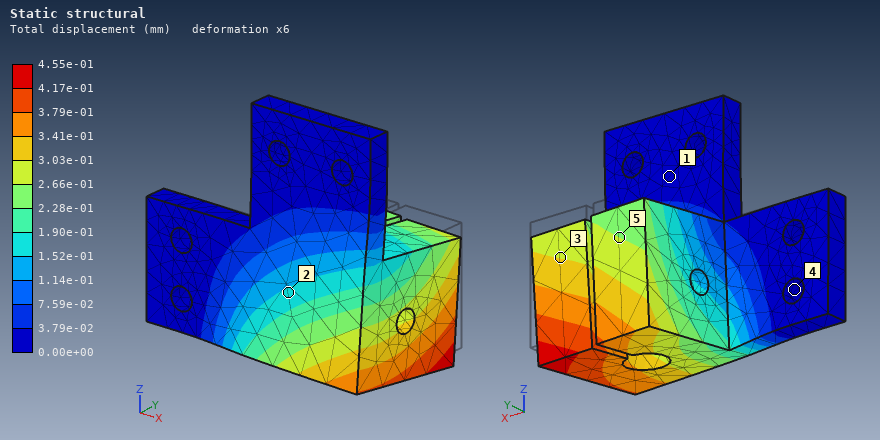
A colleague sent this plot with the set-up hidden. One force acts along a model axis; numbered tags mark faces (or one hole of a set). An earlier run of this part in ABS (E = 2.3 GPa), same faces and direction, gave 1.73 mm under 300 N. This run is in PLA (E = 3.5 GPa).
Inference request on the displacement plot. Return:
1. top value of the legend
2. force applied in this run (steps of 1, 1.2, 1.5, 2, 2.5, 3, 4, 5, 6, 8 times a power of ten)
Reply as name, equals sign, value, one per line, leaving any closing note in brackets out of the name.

top value of the legend = 4.55e-01 mm
force applied in this run = 120 N
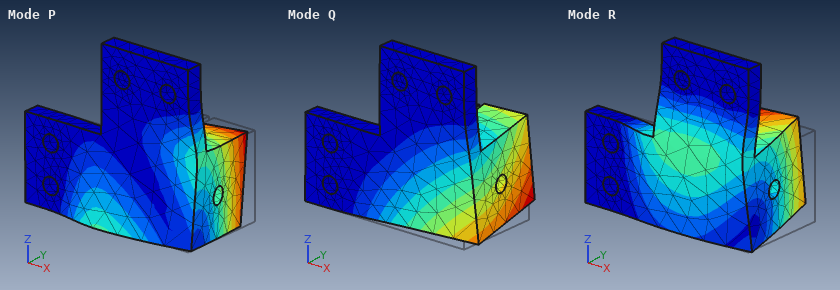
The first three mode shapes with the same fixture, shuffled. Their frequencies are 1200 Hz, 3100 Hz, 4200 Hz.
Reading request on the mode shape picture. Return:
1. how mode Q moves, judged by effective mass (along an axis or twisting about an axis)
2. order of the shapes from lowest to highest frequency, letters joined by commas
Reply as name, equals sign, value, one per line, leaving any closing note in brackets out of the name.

how mode Q moves, judged by effective mass = along Y
order of the shapes from lowest to highest frequency, letters joined by commas = Q, P, R
